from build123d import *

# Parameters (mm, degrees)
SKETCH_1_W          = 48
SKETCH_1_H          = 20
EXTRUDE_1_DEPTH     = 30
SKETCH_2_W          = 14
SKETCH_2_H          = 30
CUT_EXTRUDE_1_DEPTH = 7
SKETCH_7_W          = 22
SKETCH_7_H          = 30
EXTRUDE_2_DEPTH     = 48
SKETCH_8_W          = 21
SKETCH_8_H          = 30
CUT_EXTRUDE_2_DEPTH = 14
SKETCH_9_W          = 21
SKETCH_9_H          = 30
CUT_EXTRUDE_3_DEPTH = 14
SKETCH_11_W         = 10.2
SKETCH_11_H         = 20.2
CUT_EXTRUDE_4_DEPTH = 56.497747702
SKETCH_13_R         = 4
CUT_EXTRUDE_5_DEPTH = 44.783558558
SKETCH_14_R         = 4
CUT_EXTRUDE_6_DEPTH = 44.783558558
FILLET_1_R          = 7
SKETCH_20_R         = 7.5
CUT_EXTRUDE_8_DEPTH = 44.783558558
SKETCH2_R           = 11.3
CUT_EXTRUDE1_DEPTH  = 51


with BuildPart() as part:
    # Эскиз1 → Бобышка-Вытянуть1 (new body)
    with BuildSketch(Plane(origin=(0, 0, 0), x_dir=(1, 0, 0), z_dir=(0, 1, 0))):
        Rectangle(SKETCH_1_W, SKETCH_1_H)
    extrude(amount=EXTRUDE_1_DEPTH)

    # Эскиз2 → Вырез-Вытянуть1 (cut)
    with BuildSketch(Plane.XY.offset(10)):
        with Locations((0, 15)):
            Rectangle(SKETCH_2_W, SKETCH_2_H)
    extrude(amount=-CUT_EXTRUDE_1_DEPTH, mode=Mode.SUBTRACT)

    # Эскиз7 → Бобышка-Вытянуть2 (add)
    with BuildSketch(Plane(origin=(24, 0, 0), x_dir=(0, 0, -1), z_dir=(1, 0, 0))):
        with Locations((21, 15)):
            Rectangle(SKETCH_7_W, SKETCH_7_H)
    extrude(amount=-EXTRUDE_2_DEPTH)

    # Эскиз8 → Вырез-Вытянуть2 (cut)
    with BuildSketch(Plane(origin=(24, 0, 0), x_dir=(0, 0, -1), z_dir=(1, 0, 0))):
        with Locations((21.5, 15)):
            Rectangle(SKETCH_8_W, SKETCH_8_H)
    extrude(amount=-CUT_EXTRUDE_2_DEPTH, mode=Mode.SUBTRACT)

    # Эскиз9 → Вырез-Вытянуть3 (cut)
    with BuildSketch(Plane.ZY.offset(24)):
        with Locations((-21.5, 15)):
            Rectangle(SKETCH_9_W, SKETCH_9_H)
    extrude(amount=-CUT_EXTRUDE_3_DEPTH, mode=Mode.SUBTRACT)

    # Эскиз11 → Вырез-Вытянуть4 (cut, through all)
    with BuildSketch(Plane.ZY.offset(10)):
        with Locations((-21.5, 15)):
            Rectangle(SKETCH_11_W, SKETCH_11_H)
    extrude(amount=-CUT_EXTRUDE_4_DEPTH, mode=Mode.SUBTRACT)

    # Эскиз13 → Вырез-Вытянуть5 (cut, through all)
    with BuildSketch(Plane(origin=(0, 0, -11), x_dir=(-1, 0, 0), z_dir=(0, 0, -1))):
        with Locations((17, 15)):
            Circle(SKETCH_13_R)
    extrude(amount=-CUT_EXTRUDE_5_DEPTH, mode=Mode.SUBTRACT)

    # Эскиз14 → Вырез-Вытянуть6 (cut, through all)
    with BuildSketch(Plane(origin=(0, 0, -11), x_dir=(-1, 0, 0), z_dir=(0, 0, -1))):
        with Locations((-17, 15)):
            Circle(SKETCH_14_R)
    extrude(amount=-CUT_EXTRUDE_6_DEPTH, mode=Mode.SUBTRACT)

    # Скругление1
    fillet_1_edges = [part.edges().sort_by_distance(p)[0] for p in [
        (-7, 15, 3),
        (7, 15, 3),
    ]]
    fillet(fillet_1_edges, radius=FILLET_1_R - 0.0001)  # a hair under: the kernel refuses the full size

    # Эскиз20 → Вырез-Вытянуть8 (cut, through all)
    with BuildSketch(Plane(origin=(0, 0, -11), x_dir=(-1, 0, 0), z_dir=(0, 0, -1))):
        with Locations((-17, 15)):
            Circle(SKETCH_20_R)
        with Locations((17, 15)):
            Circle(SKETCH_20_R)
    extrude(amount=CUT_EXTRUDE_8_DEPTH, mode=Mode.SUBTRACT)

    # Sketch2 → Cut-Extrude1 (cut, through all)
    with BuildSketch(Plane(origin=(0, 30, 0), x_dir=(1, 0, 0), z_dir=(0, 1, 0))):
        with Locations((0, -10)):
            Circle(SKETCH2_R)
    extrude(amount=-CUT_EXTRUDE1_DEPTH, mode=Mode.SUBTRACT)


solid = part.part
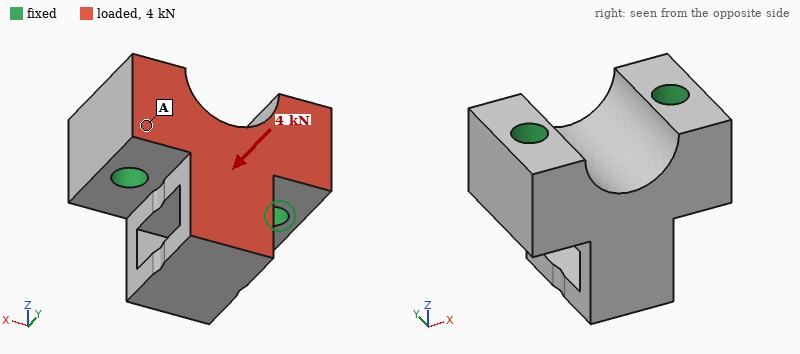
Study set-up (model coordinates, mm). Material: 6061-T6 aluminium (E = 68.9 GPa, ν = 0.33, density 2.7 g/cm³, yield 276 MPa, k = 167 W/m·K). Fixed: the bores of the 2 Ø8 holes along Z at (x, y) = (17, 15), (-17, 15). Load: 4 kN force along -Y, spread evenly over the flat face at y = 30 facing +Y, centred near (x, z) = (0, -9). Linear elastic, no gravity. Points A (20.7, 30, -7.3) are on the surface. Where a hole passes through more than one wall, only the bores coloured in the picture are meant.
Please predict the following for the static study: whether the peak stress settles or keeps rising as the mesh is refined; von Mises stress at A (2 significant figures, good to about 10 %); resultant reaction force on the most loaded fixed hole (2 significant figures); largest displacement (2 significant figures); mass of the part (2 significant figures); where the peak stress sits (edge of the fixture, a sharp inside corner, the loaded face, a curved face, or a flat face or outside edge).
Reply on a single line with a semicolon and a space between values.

keeps rising; 4.1 MPa; 2.0 kN; 21 µm; 82 g; edge of the fixture
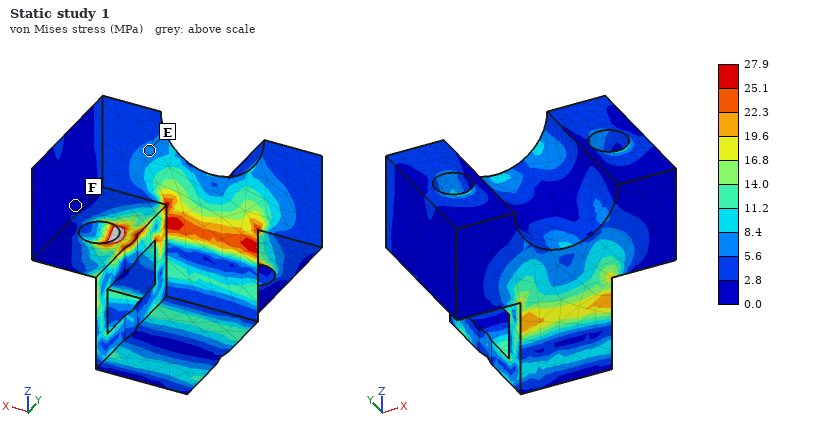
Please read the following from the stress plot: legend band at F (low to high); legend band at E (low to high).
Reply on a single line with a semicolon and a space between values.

0.0 to 2.8 MPa; 5.6 to 8.4 MPa
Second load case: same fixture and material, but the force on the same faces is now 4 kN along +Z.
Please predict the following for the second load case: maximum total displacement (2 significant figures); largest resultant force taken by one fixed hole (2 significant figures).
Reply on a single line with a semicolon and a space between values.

17 µm; 2.1 kN
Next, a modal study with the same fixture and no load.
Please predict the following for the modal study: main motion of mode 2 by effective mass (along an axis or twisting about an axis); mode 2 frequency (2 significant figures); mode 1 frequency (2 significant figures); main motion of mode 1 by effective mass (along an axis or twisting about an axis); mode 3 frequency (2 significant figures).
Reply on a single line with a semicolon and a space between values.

along X; 14 kHz; 9800 Hz; along Y; 20 kHz
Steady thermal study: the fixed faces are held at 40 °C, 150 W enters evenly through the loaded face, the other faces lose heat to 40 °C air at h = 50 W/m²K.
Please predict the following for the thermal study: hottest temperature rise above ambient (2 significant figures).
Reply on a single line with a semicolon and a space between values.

32 K
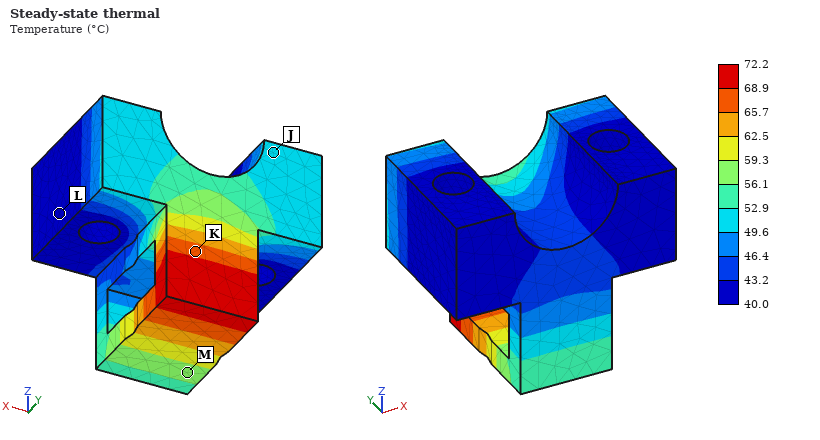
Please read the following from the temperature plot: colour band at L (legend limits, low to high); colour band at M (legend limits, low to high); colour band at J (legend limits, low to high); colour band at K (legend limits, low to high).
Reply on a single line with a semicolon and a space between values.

40.0 to 43.2 °C; 56.1 to 59.3 °C; 49.6 to 52.9 °C; 65.7 to 68.9 °C
